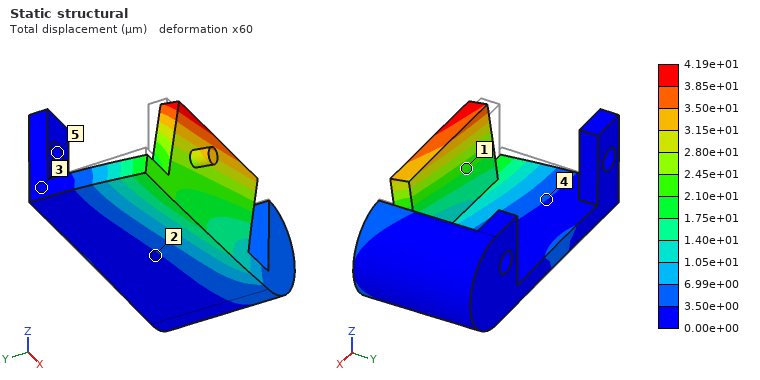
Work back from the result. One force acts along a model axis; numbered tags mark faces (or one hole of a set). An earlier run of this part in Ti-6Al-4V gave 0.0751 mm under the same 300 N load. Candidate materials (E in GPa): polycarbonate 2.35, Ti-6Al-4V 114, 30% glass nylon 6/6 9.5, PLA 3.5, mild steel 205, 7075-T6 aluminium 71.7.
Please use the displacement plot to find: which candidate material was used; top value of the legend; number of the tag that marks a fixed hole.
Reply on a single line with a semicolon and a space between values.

mild steel; 4.19e+01 µm; 5
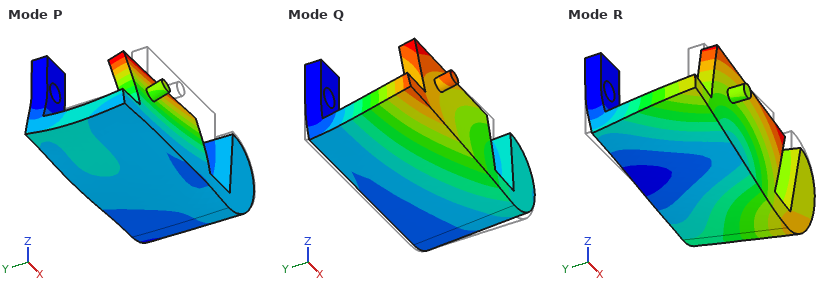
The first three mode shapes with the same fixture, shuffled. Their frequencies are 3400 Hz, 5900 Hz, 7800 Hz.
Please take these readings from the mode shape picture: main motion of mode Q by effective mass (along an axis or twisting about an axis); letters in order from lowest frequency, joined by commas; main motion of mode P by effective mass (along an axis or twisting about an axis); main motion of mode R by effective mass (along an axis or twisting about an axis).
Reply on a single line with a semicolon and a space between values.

along Z; Q, R, P; along Y; along X
